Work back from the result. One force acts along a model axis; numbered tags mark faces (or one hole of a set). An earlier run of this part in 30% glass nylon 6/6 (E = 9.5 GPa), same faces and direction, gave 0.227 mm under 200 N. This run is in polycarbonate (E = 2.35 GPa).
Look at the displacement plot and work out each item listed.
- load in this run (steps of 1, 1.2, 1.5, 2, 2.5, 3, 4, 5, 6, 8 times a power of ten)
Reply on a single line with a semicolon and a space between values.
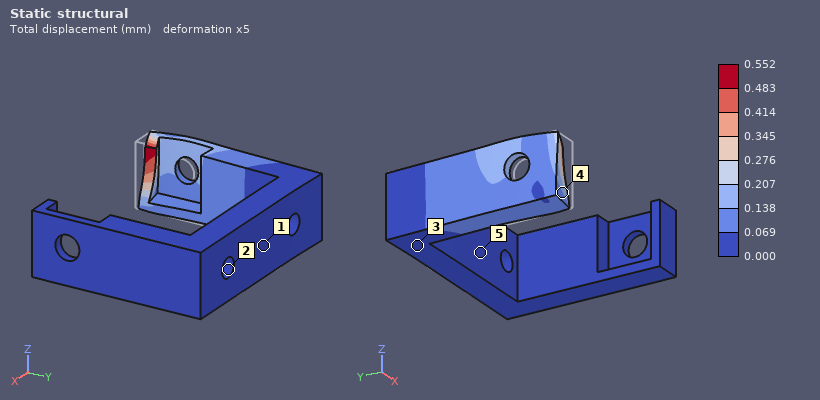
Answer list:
120 N
